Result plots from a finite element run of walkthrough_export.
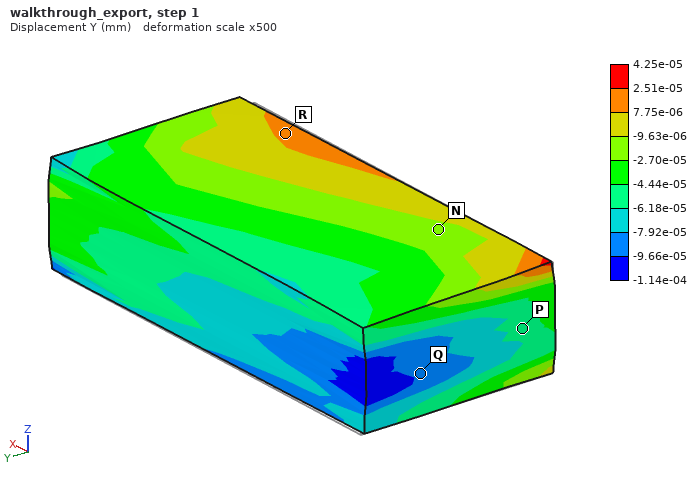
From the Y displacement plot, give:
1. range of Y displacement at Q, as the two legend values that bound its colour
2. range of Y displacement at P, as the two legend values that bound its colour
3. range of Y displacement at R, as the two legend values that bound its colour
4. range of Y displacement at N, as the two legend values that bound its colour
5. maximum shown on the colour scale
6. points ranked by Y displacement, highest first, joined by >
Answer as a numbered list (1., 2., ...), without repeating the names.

1. -9.66e-05 to -7.92e-05 mm
2. -6.18e-05 to -4.44e-05 mm
3. 7.75e-06 to 2.51e-05 mm
4. -2.70e-05 to -9.63e-06 mm
5. 4.25e-05 mm
6. R > N > P > Q
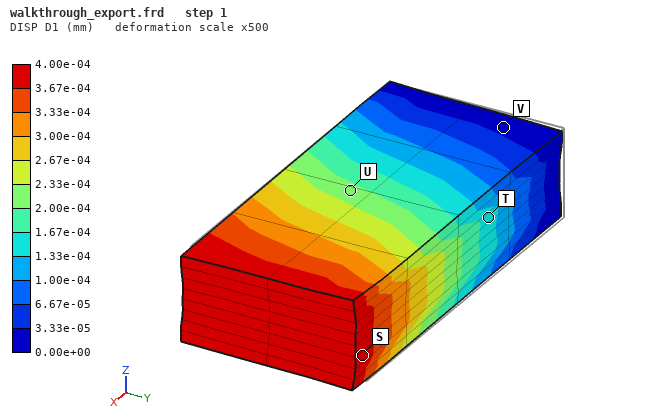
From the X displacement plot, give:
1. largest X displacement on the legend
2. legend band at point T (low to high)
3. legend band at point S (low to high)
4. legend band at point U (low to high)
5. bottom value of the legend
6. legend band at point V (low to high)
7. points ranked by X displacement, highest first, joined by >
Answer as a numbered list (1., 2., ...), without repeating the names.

1. 4.00e-04 mm
2. 1.33e-04 to 1.67e-04 mm
3. 3.67e-04 to 4.00e-04 mm
4. 2.00e-04 to 2.33e-04 mm
5. 0.00e+00 mm
6. 0.00e+00 to 3.33e-05 mm
7. S > U > T > V
